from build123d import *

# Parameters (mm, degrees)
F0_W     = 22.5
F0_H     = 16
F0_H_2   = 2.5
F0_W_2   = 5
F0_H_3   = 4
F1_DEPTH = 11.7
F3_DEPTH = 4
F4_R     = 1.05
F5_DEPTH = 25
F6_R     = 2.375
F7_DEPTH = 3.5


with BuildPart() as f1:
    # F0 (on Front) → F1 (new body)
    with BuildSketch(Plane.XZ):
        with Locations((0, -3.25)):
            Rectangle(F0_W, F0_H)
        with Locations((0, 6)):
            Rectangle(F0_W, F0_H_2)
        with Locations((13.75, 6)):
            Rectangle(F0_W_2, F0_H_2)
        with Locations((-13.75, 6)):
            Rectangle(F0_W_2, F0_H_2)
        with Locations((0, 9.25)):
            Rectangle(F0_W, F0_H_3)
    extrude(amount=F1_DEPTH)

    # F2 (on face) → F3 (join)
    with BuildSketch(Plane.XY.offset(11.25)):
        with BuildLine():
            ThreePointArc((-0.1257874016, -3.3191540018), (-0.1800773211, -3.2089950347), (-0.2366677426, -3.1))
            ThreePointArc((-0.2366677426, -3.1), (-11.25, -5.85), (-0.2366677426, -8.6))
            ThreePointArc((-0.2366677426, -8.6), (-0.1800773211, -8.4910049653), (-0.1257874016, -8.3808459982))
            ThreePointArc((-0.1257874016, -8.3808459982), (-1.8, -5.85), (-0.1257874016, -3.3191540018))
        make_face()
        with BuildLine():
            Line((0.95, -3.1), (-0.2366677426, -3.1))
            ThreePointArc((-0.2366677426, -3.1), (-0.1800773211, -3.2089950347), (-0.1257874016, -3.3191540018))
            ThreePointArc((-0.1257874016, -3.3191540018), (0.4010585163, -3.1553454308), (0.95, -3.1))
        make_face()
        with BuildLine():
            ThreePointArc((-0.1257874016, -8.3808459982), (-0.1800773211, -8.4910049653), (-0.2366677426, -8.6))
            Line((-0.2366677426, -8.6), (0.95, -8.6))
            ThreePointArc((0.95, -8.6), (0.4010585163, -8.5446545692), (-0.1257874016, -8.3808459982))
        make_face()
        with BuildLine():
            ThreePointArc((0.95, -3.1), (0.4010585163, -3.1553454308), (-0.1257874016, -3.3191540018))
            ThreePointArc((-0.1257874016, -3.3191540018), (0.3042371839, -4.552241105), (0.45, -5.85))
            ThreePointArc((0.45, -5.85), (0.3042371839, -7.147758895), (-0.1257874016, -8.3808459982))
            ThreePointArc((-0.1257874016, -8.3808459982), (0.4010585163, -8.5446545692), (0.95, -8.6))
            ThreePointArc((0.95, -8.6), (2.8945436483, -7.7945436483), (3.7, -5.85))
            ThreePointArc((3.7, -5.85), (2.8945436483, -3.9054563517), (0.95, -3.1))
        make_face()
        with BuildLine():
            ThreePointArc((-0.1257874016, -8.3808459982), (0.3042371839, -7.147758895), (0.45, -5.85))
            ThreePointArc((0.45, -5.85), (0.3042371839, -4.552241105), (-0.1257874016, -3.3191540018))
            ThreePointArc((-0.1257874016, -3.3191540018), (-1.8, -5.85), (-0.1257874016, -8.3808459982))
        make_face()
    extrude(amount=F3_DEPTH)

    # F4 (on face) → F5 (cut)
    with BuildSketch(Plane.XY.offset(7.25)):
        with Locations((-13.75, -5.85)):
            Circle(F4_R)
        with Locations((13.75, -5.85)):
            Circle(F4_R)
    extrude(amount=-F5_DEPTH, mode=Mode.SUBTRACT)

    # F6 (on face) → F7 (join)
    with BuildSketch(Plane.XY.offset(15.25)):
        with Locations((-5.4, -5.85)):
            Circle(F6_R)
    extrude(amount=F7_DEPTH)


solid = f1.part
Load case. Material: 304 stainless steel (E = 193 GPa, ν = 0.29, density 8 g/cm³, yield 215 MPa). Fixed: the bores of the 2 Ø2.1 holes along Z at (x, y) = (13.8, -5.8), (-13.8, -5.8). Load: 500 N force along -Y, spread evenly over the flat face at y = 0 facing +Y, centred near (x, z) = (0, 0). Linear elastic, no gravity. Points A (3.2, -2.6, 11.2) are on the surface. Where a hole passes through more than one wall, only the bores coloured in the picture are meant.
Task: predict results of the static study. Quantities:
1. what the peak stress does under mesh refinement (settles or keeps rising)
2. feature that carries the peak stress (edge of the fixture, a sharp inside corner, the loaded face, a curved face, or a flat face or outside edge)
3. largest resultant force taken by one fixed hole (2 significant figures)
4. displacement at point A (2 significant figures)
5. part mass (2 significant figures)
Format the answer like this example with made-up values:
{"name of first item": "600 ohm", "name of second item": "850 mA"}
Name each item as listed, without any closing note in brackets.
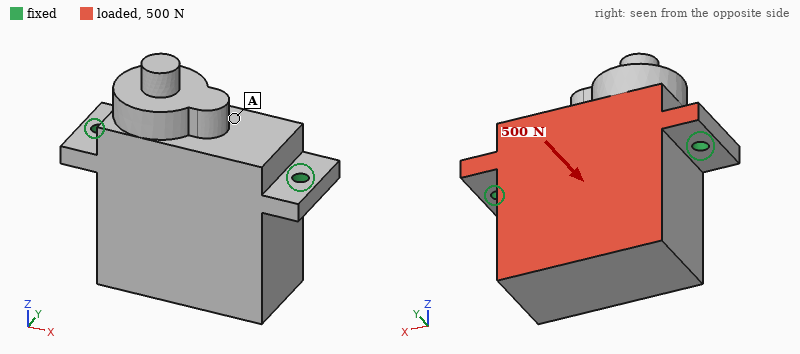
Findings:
{"what the peak stress does under mesh refinement": "keeps rising", "feature that carries the peak stress": "edge of the fixture", "largest resultant force taken by one fixed hole": "250 N", "displacement at point A": "5.5 µm", "part mass": "54 g"}
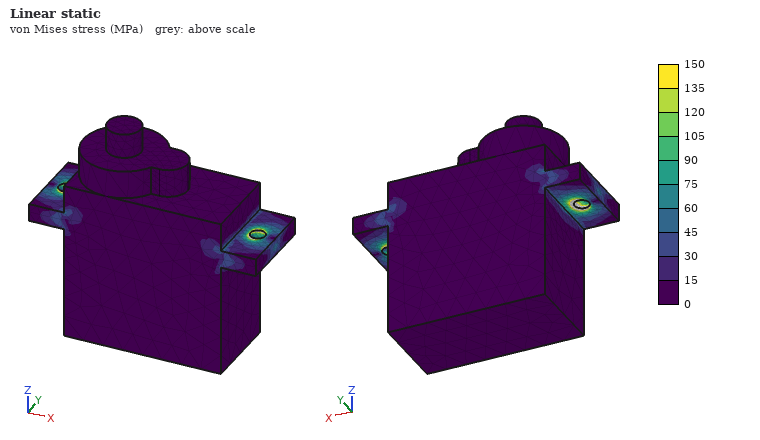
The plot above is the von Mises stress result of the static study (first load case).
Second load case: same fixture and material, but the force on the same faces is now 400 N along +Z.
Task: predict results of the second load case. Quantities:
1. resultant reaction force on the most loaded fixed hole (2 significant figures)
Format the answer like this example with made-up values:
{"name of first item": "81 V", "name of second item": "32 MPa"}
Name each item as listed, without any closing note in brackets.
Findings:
{"resultant reaction force on the most loaded fixed hole": "200 N"}
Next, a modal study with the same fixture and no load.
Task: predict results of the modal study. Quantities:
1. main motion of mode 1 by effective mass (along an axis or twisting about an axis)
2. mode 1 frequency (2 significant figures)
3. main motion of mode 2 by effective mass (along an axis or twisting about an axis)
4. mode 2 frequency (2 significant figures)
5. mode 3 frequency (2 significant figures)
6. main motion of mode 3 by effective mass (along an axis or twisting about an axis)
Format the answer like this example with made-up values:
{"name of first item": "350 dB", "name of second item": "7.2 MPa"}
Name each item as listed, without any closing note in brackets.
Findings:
{"main motion of mode 1 by effective mass": "along Y", "mode 1 frequency": "3900 Hz", "main motion of mode 2 by effective mass": "along Z", "mode 2 frequency": "15 kHz", "mode 3 frequency": "16 kHz", "main motion of mode 3 by effective mass": "along X"}
